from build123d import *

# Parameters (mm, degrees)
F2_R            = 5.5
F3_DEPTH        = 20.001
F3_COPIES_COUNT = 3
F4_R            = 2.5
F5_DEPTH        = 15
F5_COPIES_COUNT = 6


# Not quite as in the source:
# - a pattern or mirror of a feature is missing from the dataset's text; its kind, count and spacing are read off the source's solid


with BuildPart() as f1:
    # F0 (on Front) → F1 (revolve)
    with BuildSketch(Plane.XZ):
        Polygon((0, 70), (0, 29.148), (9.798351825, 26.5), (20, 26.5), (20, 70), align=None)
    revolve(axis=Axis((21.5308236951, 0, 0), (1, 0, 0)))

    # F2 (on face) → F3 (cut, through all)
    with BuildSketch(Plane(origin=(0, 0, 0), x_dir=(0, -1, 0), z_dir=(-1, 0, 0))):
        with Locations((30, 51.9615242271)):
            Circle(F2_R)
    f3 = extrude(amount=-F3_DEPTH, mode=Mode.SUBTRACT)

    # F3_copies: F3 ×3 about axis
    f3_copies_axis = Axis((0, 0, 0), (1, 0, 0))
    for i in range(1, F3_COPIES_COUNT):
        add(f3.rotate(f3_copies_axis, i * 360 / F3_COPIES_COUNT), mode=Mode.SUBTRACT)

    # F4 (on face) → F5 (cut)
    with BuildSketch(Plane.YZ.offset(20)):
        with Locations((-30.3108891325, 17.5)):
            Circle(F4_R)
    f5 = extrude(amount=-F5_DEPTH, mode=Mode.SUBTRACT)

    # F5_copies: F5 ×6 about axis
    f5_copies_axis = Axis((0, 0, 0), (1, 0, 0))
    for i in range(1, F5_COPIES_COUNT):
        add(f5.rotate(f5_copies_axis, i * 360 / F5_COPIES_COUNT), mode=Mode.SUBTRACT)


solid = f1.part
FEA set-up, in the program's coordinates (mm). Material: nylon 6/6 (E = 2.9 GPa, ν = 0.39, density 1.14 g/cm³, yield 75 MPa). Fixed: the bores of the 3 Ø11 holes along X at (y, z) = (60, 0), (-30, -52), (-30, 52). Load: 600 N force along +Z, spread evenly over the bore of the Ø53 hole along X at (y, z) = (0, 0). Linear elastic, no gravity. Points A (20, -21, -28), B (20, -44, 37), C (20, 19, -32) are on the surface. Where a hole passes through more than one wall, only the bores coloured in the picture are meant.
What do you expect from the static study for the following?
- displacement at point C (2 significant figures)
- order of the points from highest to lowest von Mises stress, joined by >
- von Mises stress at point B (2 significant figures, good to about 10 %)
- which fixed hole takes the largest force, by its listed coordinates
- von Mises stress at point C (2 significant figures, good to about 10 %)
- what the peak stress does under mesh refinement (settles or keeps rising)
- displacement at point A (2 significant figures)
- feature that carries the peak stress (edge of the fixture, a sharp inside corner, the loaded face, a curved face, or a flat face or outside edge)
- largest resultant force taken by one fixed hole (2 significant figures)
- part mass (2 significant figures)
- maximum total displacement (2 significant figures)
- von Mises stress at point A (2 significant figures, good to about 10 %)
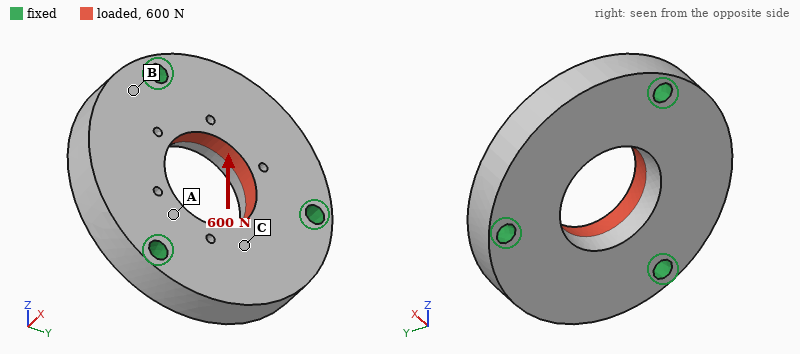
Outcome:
8.4 µm
A > C > B
0.12 MPa
(60, 0)
0.27 MPa
keeps rising
3.5 µm
edge of the fixture
220 N
290 g
9.7 µm
0.42 MPa
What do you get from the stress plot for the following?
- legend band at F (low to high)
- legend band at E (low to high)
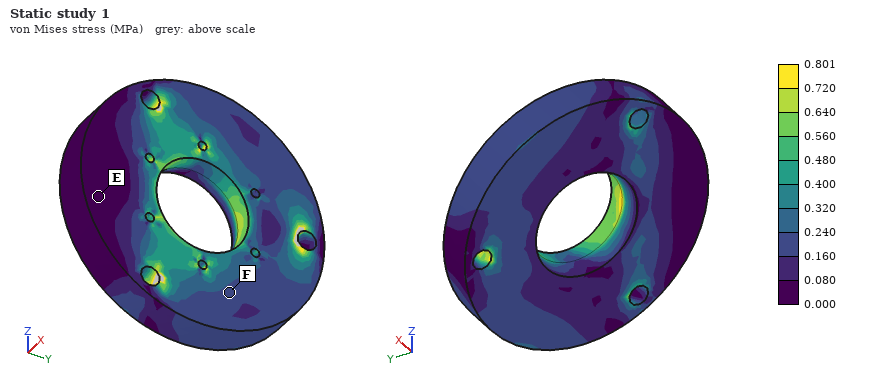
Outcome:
0.160 to 0.240 MPa
0.000 to 0.080 MPa
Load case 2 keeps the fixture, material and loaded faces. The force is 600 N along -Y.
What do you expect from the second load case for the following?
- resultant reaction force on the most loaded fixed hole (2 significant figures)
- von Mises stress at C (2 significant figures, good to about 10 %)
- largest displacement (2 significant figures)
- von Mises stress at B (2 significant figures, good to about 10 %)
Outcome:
210 N
0.19 MPa
11 µm
0.32 MPa
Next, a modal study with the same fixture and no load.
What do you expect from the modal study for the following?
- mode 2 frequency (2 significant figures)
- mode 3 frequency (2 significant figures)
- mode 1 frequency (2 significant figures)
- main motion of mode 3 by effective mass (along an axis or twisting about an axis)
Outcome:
1800 Hz
2100 Hz
1800 Hz
along X
